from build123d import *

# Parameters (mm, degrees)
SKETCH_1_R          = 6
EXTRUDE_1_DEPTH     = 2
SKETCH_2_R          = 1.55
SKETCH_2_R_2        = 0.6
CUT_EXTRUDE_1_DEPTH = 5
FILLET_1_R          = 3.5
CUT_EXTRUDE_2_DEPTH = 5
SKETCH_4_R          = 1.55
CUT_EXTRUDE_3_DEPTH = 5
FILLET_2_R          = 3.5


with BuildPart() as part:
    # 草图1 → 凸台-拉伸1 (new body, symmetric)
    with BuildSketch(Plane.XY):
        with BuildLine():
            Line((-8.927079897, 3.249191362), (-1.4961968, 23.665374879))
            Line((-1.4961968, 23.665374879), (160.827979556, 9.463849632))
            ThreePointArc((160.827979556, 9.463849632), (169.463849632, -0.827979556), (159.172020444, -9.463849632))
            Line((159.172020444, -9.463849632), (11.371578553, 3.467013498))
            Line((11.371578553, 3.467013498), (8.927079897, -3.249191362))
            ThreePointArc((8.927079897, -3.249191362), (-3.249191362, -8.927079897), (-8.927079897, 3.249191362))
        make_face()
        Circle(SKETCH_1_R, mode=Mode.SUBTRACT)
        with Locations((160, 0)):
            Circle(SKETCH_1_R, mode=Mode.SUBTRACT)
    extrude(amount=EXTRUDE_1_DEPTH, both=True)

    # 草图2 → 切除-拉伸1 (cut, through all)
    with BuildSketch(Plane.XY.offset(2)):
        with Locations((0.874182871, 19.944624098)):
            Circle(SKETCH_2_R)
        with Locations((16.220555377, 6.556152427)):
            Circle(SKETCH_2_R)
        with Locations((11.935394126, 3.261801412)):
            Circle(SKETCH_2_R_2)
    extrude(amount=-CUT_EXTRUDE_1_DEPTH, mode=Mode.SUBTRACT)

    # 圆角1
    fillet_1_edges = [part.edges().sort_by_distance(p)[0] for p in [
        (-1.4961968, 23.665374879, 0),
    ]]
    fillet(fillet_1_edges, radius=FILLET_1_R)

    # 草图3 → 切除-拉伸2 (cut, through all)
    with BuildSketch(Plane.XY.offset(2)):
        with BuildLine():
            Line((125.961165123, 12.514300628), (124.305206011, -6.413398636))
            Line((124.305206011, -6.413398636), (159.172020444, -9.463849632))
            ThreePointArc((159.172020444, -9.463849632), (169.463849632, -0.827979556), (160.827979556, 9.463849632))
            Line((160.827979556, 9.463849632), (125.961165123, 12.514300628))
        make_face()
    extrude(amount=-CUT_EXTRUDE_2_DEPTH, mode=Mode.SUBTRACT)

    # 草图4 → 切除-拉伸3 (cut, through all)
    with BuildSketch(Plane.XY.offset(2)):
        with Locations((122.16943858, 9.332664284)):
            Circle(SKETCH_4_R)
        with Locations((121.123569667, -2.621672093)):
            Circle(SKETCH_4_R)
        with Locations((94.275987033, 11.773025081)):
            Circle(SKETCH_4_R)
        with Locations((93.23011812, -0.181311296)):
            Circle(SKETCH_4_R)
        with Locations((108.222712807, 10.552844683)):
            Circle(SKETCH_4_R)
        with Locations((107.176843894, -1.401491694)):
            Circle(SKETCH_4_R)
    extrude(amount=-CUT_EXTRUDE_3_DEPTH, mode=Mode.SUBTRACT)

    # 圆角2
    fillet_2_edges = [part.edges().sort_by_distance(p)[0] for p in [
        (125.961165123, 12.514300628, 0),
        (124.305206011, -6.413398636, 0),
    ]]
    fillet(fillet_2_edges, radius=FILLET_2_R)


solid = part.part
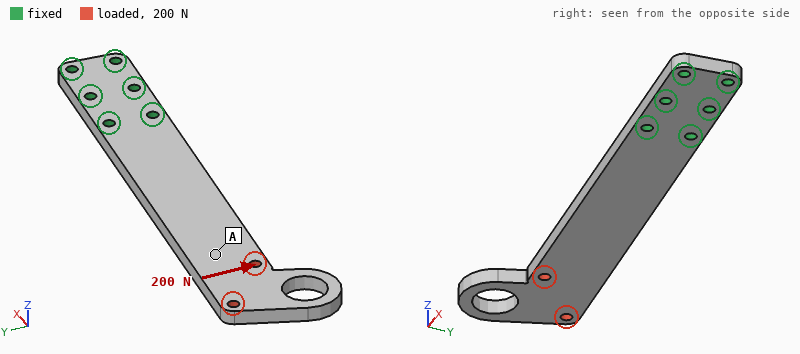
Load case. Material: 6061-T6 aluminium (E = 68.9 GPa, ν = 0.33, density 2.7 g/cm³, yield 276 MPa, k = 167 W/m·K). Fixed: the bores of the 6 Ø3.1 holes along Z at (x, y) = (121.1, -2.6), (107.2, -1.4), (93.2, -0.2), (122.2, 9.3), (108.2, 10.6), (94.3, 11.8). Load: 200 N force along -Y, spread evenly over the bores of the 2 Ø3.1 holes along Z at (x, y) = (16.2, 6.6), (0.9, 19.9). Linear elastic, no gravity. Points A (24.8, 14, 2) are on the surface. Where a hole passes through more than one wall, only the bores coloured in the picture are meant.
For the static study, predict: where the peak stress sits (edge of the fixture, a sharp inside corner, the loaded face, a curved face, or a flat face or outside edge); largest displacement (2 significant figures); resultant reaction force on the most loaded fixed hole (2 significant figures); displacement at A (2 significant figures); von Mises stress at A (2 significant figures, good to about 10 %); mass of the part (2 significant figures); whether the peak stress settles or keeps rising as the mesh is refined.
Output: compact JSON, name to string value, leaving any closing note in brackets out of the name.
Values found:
{"where the peak stress sits": "edge of the fixture", "largest displacement": "0.36 mm", "resultant reaction force on the most loaded fixed hole": "1.2 kN", "displacement at A": "0.20 mm", "von Mises stress at A": "6.8 MPa", "mass of the part": "27 g", "whether the peak stress settles or keeps rising as the mesh is refined": "keeps rising"}
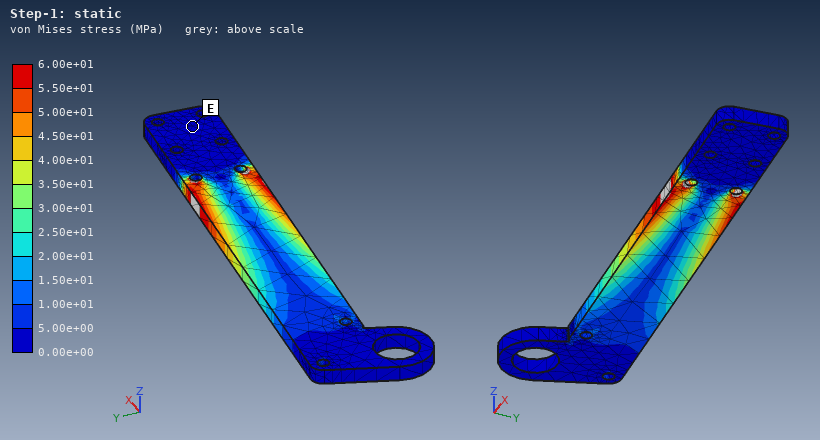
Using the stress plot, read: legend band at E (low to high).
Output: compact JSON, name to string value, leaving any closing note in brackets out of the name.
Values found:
{"legend band at E": "0.00e+00 to 5.00e+00 MPa"}
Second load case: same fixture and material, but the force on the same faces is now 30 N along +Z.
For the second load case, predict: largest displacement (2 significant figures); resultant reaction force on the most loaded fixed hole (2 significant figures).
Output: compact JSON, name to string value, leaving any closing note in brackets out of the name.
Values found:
{"largest displacement": "1.1 mm", "resultant reaction force on the most loaded fixed hole": "30 N"}
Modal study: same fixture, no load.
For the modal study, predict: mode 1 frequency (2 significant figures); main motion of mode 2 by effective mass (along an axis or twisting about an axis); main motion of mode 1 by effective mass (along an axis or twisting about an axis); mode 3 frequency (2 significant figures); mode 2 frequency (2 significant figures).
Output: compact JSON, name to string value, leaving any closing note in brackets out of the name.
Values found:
{"mode 1 frequency": "310 Hz", "main motion of mode 2 by effective mass": "along Y", "main motion of mode 1 by effective mass": "along Z", "mode 3 frequency": "1800 Hz", "mode 2 frequency": "1400 Hz"}
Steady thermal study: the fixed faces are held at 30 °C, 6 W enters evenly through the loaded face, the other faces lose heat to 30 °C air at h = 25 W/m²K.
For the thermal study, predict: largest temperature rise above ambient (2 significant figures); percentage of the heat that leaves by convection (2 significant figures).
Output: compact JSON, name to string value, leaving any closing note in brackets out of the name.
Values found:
{"largest temperature rise above ambient": "31 K", "percentage of the heat that leaves by convection": "35 %"}
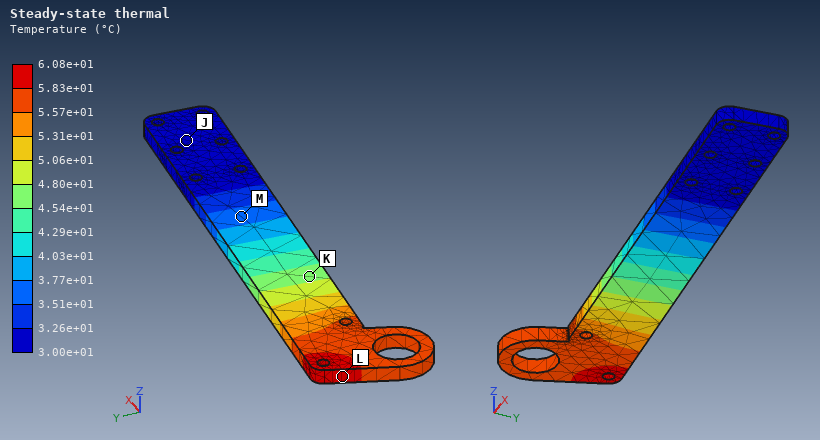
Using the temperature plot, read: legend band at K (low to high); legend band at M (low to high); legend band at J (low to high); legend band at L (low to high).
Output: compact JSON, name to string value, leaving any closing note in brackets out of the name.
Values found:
{"legend band at K": "4.54e+01 to 4.80e+01 °C", "legend band at M": "3.51e+01 to 3.77e+01 °C", "legend band at J": "3.00e+01 to 3.26e+01 °C", "legend band at L": "5.83e+01 to 6.08e+01 °C"}
